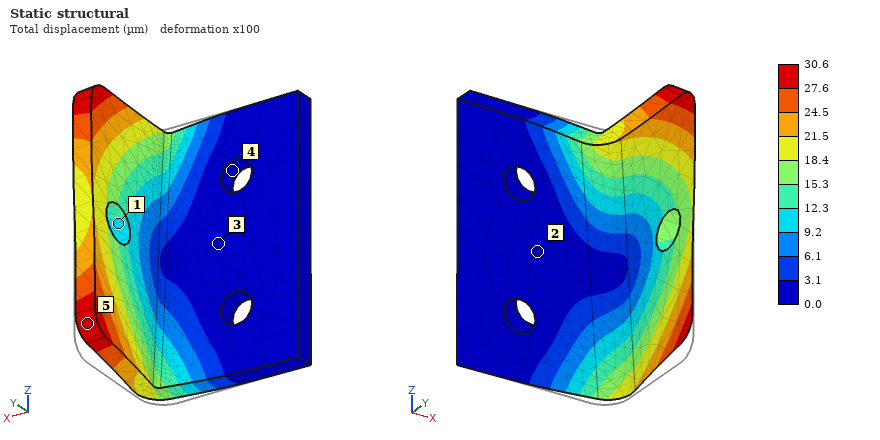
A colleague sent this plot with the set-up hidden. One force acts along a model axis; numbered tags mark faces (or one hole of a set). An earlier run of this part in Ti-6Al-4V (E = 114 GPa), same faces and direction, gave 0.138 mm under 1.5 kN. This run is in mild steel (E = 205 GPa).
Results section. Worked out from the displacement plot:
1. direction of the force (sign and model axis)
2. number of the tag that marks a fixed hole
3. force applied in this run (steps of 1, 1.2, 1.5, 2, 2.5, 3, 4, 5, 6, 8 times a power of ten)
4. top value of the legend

+Z
4
600 N
30.6 µm
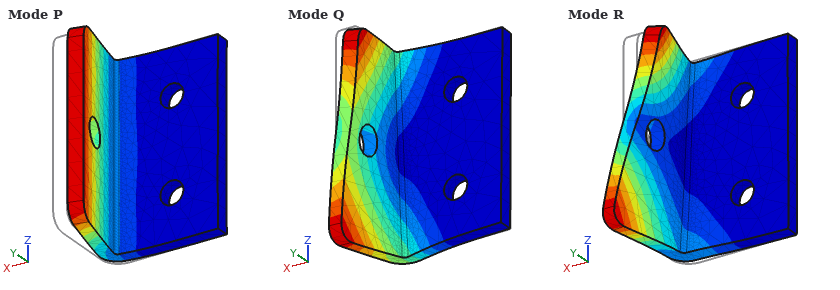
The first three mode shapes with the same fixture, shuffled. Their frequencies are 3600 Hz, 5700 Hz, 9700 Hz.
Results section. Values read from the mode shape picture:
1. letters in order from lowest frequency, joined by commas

P, Q, R
